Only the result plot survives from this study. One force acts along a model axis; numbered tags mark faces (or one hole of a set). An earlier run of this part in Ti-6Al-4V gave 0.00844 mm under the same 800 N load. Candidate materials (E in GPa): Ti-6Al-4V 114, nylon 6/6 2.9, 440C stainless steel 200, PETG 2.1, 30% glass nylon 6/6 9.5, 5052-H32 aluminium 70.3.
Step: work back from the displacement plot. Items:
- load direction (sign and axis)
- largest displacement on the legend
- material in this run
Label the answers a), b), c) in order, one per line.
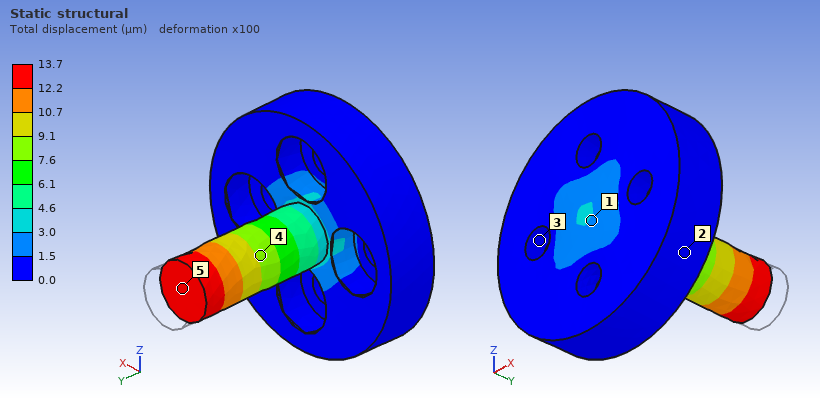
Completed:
a) -Y
b) 13.7 µm
c) 5052-H32 aluminium
